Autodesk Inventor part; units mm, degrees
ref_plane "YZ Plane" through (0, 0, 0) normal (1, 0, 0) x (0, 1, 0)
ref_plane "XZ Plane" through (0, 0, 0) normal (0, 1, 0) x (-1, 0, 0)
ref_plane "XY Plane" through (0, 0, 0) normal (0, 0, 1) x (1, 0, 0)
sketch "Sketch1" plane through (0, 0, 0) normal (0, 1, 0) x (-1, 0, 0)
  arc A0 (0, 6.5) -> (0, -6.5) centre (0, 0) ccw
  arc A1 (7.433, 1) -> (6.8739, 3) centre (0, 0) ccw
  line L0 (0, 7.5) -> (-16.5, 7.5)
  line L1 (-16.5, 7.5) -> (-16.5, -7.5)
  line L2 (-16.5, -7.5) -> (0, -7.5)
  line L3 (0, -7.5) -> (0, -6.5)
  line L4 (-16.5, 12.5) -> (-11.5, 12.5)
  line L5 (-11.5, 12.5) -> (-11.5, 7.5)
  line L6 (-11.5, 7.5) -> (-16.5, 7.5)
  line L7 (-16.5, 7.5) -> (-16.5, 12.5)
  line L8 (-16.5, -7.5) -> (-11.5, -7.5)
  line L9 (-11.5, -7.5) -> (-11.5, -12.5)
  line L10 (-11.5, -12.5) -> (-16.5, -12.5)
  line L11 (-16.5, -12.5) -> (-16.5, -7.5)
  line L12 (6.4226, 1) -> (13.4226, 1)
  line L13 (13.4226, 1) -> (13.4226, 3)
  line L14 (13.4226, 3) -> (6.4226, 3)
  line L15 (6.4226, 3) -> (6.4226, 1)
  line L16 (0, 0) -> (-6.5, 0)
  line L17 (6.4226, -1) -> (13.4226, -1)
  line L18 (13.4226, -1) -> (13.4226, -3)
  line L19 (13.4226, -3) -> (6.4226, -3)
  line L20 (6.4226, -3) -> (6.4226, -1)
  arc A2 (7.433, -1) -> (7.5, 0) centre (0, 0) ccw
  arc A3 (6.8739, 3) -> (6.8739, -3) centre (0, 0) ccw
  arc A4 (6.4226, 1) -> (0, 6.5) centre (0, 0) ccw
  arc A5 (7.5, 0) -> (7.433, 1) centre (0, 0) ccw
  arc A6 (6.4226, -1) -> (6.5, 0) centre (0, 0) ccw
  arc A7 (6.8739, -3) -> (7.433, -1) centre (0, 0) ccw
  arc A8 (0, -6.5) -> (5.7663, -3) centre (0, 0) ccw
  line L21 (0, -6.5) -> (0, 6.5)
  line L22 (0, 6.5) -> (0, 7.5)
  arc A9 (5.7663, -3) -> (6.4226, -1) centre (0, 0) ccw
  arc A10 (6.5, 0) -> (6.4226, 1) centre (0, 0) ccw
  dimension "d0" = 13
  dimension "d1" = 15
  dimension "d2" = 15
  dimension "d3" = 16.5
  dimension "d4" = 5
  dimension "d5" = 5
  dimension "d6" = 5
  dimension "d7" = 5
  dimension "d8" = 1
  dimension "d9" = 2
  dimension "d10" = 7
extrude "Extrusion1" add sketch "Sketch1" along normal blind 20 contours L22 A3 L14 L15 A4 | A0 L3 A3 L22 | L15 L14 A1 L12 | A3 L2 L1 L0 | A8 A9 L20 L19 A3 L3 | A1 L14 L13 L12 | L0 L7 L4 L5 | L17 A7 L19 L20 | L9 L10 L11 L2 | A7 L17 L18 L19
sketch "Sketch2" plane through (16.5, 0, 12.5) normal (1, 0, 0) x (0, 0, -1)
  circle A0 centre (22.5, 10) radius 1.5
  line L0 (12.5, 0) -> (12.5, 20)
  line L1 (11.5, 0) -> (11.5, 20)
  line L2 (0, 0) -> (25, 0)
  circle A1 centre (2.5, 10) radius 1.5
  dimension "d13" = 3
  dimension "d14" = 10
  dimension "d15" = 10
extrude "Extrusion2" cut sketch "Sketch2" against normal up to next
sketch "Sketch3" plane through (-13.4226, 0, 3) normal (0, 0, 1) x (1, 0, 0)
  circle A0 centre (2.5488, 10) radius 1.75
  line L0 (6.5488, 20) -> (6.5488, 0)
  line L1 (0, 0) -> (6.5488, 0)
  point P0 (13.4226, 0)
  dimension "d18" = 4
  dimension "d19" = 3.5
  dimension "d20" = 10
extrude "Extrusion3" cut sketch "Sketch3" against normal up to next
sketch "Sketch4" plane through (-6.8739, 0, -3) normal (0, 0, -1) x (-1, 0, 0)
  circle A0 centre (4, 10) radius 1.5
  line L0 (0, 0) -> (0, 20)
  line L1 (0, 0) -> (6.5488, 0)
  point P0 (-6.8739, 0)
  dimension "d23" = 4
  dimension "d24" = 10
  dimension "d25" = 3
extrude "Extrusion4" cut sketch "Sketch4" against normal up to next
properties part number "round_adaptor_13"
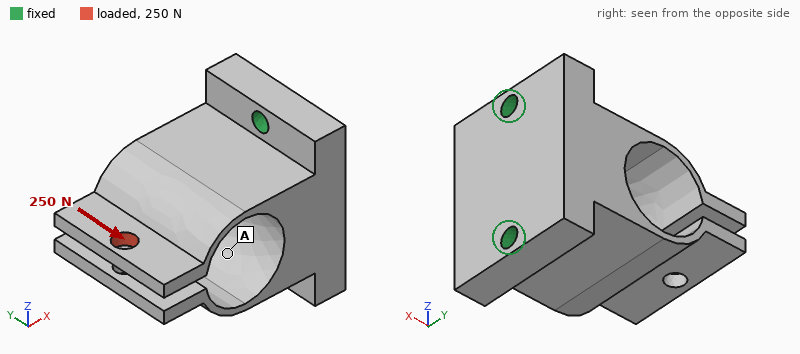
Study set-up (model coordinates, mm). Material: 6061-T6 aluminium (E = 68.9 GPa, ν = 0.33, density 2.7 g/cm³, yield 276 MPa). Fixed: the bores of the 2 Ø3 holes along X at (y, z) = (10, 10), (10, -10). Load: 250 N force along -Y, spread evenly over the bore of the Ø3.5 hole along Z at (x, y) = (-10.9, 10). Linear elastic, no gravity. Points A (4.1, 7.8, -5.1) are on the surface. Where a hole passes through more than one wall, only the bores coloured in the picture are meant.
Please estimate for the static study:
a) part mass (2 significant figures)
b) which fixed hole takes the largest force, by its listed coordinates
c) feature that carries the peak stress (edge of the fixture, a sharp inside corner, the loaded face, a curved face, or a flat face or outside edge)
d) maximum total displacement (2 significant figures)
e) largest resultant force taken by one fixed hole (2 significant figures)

15 g
(10, 10)
a flat face or outside edge
0.11 mm
140 N
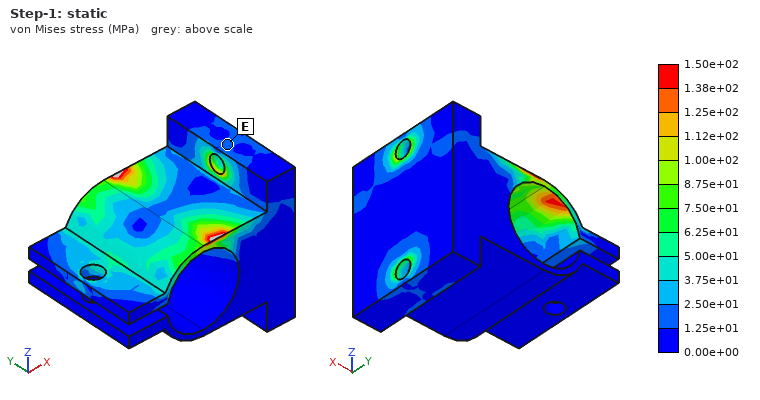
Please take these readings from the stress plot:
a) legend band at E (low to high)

1.25e+01 to 2.50e+01 MPa
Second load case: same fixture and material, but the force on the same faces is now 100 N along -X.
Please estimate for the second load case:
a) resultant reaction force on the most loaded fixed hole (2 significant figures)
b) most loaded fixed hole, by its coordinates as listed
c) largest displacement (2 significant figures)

64 N
(10, 10)
0.39 mm
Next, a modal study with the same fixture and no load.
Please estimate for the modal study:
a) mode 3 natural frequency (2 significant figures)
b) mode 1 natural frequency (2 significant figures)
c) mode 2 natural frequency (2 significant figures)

5700 Hz
2200 Hz
2200 Hz
